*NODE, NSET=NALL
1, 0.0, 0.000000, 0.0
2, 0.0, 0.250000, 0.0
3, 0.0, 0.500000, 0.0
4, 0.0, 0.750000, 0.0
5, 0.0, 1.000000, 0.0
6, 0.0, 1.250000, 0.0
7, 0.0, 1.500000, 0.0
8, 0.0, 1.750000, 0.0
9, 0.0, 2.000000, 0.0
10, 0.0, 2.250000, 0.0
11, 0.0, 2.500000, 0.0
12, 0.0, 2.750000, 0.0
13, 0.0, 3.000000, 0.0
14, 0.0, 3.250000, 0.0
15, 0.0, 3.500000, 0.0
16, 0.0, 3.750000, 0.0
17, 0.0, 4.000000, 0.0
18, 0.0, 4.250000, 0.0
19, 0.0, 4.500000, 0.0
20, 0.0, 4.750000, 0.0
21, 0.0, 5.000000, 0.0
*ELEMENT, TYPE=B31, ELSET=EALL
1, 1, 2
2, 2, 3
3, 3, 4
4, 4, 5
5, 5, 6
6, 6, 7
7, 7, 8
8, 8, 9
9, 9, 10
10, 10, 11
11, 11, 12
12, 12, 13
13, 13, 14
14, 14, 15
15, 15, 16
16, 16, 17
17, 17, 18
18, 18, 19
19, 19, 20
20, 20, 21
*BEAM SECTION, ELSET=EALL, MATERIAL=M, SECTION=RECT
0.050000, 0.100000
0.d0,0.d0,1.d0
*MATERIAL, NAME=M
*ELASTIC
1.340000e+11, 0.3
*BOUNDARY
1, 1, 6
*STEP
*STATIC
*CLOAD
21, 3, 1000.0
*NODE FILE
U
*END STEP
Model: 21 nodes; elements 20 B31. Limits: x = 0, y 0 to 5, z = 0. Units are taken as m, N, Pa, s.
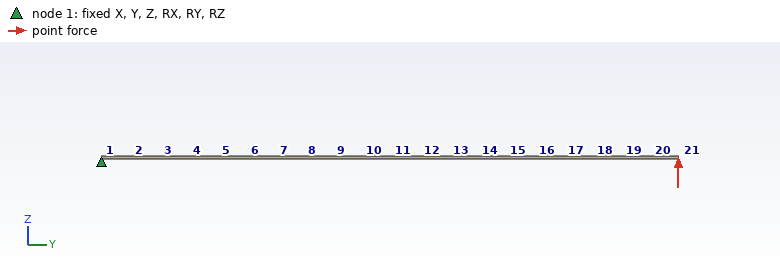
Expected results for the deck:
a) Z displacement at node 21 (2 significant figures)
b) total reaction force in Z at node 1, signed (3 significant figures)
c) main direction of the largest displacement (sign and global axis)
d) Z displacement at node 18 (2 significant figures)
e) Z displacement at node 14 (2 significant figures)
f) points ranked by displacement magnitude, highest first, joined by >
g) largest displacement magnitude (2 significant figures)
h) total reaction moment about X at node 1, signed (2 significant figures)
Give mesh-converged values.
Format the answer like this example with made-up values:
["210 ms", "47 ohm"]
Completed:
["0.30 m", "-1000 N", "+Z", "0.23 m", "0.15 m", "node 21 > node 18 > node 16 > node 14 > node 7", "0.30 m", "-5000 N·m"]
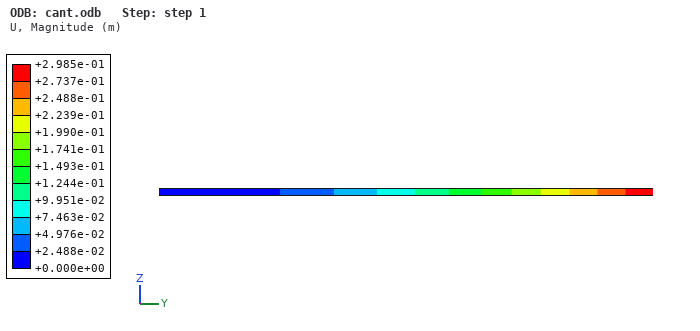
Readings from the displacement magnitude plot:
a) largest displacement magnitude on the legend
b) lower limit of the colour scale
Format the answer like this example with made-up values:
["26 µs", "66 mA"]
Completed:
["+2.985e-01 m", "+0.000e+00 m"]
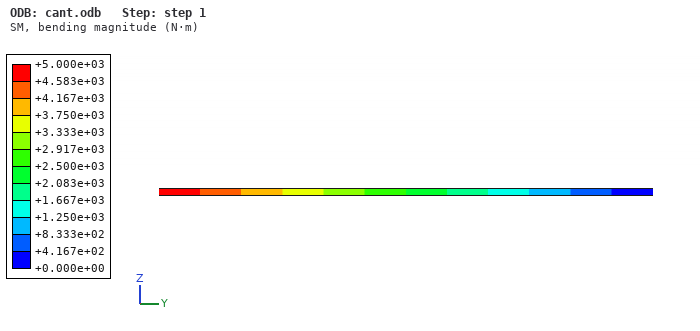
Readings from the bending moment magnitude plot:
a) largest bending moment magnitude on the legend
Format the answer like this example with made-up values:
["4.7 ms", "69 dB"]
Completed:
["+5.000e+03 N·m"]
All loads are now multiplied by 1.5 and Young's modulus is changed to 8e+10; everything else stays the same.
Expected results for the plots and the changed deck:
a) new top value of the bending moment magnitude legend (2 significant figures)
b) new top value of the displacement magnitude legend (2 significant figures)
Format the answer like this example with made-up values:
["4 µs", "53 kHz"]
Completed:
["7500 N·m", "0.75 m"]
